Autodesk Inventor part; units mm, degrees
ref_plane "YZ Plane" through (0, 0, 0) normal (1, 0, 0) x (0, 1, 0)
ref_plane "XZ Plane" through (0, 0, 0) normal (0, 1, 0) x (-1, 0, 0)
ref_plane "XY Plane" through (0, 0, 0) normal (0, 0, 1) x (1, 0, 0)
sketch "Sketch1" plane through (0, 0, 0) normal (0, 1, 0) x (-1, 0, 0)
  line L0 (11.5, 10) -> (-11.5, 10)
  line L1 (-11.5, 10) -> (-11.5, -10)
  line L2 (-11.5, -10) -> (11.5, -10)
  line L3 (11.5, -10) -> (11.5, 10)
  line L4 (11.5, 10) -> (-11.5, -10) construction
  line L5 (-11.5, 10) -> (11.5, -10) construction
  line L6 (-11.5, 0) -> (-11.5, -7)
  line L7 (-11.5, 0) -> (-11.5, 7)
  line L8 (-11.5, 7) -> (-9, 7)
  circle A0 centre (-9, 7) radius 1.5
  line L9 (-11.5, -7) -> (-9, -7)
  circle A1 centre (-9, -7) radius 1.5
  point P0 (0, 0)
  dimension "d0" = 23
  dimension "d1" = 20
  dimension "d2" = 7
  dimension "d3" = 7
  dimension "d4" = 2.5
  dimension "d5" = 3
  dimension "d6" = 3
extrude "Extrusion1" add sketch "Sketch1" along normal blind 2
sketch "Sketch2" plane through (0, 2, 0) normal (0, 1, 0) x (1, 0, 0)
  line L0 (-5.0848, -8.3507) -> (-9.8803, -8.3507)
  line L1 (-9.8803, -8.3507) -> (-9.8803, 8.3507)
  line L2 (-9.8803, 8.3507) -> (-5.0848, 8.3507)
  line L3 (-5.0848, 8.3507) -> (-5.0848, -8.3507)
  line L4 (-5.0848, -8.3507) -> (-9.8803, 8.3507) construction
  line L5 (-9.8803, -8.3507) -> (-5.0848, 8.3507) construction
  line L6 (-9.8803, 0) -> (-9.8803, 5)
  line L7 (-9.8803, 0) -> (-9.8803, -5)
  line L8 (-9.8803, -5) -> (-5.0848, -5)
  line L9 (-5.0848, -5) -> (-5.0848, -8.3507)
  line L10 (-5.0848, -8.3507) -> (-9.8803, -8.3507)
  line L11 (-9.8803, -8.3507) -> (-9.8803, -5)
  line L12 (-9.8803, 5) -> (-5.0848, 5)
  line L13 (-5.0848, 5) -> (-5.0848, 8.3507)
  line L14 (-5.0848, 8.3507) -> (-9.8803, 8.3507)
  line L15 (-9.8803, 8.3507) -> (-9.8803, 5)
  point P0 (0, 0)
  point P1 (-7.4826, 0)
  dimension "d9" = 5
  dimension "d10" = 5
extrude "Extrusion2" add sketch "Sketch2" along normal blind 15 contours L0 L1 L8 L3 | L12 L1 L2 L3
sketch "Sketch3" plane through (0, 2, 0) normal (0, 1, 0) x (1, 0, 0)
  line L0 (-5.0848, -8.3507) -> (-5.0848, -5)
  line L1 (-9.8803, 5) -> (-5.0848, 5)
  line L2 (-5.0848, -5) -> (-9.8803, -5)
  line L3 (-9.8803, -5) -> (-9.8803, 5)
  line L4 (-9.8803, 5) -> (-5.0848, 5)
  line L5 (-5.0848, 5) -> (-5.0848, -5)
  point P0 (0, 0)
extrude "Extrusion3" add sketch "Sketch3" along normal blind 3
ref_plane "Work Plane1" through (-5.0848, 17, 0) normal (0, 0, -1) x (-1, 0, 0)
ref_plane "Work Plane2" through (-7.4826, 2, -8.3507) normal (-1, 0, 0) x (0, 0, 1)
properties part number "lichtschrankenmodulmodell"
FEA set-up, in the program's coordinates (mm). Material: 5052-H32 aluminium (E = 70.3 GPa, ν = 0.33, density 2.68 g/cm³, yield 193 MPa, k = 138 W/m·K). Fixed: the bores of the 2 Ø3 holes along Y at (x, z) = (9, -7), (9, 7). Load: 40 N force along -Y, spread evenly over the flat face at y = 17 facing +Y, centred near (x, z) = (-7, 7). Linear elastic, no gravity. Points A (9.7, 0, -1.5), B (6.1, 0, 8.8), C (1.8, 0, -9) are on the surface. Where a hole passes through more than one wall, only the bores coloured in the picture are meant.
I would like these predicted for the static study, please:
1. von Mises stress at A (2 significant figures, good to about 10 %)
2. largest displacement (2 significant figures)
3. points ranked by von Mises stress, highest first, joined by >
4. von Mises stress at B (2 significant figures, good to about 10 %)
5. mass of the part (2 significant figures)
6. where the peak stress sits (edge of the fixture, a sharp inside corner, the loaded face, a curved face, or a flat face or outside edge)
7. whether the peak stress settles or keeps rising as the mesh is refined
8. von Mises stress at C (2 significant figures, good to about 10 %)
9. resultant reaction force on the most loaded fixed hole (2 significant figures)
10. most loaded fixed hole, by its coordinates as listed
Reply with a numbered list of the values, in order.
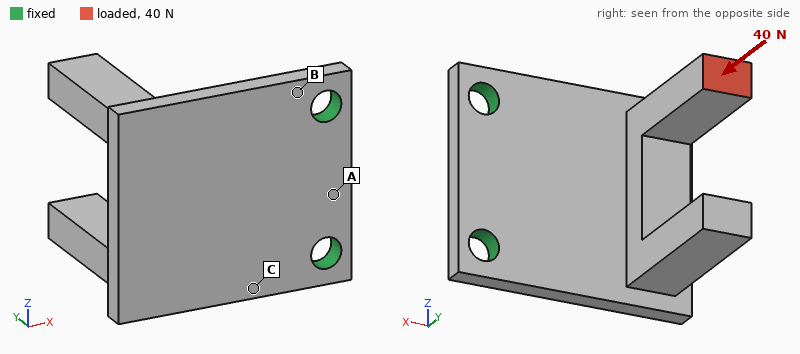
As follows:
1. 11 MPa
2. 0.12 mm
3. B > C > A
4. 56 MPa
5. 4.1 g
6. edge of the fixture
7. keeps rising
8. 28 MPa
9. 38 N
10. (9, 7)
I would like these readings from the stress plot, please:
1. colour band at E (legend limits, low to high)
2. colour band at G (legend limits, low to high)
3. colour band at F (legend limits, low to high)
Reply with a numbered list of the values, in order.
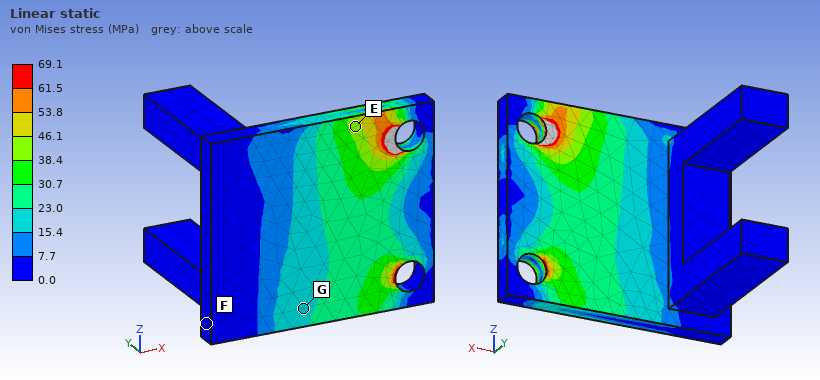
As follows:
1. 38.4 to 46.1 MPa
2. 15.4 to 23.0 MPa
3. 0.0 to 7.7 MPa
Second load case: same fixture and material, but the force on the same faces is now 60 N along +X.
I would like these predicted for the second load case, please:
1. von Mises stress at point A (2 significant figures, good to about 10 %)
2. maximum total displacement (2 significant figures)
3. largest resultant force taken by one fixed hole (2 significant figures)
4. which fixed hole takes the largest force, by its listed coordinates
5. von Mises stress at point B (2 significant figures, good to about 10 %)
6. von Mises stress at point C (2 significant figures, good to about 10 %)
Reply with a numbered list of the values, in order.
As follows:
1. 17 MPa
2. 0.33 mm
3. 58 N
4. (9, 7)
5. 73 MPa
6. 74 MPa
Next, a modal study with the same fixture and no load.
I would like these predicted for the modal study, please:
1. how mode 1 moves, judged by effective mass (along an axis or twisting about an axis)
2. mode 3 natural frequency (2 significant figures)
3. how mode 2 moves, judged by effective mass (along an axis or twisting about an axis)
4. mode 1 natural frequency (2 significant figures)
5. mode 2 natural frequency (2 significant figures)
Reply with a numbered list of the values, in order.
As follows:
1. along Y
2. 8500 Hz
3. along Z
4. 2100 Hz
5. 4600 Hz
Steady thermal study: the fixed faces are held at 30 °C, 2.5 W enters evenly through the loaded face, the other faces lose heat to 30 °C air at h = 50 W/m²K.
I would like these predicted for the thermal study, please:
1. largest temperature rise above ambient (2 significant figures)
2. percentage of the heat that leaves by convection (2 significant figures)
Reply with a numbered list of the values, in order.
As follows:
1. 23 K
2. 17 %
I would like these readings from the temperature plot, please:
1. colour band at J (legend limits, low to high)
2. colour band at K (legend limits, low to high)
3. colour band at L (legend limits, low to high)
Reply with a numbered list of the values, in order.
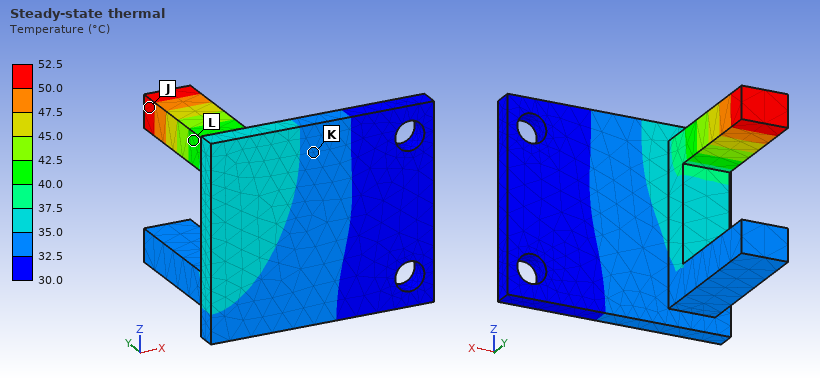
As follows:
1. 50.0 to 52.5 °C
2. 32.5 to 35.0 °C
3. 40.0 to 42.5 °C
